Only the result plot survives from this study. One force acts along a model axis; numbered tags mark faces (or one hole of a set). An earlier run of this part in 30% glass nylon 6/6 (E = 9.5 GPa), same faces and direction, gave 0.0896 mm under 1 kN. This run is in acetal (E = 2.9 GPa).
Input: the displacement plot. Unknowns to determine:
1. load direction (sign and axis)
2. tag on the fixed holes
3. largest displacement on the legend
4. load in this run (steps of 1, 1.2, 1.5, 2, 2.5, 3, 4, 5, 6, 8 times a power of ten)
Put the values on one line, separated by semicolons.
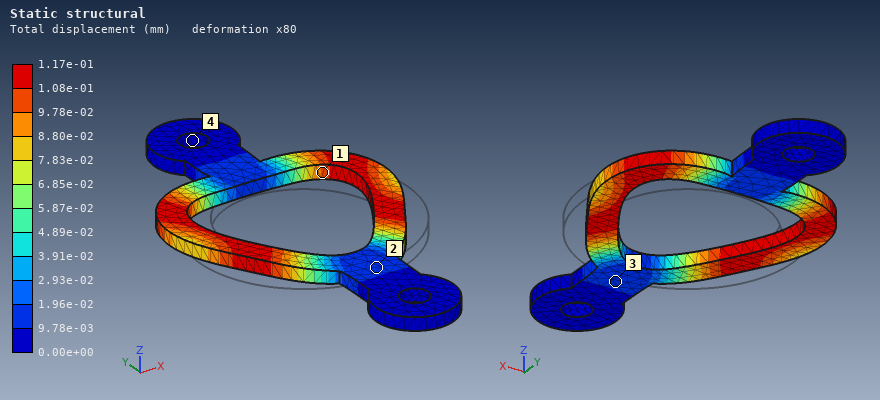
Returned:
+Y; 4; 1.17e-01 mm; 400 N
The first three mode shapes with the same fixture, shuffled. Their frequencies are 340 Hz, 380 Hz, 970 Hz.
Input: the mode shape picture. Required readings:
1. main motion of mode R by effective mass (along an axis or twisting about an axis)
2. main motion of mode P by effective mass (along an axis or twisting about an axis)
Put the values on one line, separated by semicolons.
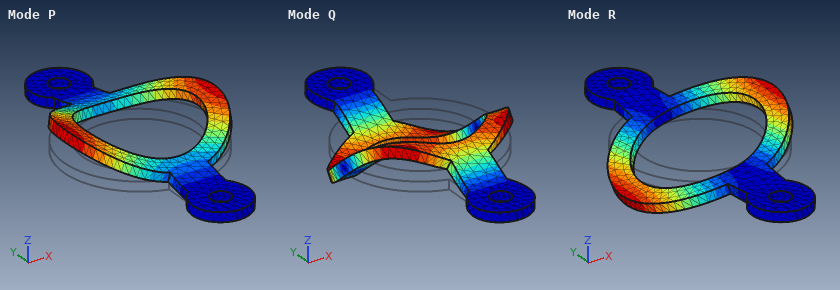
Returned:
twisting about Y; along Z
